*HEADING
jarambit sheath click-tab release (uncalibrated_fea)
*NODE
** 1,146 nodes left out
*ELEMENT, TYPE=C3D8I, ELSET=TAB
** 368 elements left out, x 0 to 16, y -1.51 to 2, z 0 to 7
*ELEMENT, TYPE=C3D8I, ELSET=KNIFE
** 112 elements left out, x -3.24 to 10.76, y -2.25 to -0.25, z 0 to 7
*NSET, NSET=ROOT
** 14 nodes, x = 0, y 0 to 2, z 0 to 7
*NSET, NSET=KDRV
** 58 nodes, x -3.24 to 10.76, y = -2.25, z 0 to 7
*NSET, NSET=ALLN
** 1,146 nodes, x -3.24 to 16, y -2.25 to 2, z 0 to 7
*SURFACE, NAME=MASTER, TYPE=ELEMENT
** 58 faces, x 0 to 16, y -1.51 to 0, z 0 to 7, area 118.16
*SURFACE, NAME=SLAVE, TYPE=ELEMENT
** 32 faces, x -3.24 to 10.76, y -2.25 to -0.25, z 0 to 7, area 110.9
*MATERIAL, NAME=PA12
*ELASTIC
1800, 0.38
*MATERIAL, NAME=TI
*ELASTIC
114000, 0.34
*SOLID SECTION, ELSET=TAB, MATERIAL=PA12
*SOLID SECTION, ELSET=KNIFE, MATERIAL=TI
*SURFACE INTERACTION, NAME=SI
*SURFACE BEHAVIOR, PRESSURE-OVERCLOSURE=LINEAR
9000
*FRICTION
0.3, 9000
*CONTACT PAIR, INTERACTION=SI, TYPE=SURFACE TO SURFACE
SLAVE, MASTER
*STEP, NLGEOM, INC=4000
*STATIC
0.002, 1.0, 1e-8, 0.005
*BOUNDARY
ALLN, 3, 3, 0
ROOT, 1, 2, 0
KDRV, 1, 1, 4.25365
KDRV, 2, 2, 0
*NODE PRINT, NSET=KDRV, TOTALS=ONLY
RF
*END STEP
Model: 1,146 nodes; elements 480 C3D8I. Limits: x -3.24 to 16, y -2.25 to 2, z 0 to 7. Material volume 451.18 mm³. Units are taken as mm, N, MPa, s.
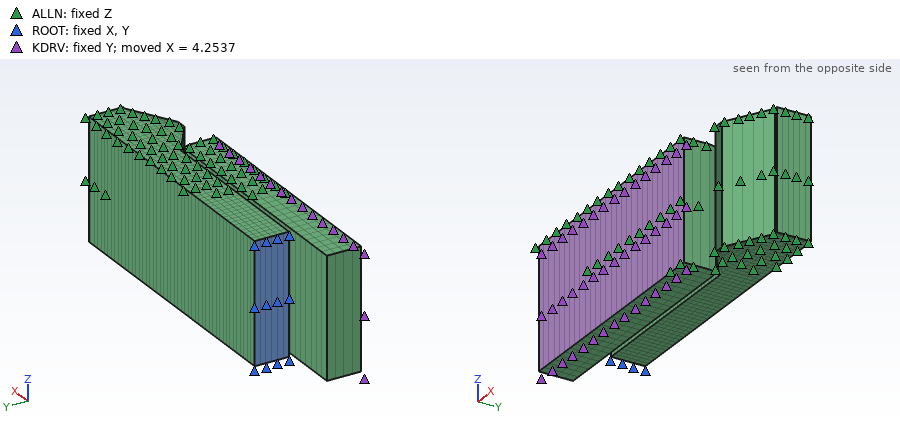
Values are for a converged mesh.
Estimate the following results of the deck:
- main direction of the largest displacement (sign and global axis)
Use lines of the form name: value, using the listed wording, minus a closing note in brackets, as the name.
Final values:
main direction of the largest displacement: +X
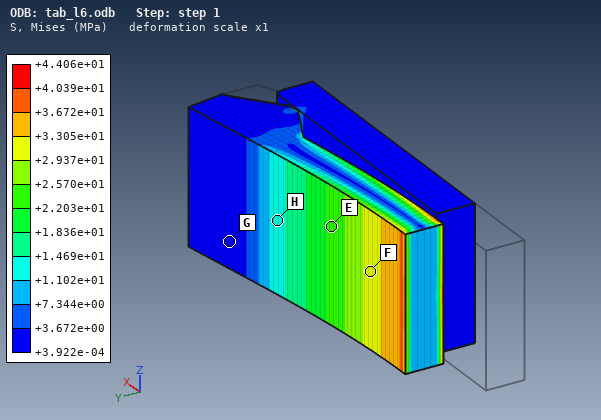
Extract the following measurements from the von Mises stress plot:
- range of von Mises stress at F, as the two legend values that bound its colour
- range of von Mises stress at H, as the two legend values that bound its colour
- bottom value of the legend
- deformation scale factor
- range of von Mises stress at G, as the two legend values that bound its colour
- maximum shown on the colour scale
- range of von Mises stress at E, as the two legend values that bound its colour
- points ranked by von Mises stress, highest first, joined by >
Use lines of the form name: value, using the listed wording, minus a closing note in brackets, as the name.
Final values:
range of von Mises stress at F, as the two legend values that bound its colour: +2.937e+01 to +3.305e+01 MPa
range of von Mises stress at H, as the two legend values that bound its colour: +1.102e+01 to +1.469e+01 MPa
bottom value of the legend: +3.922e-04 MPa
deformation scale factor: 1
range of von Mises stress at G, as the two legend values that bound its colour: +3.922e-04 to +3.672e+00 MPa
maximum shown on the colour scale: +4.406e+01 MPa
range of von Mises stress at E, as the two legend values that bound its colour: +2.203e+01 to +2.570e+01 MPa
points ranked by von Mises stress, highest first, joined by >: F > E > H > G
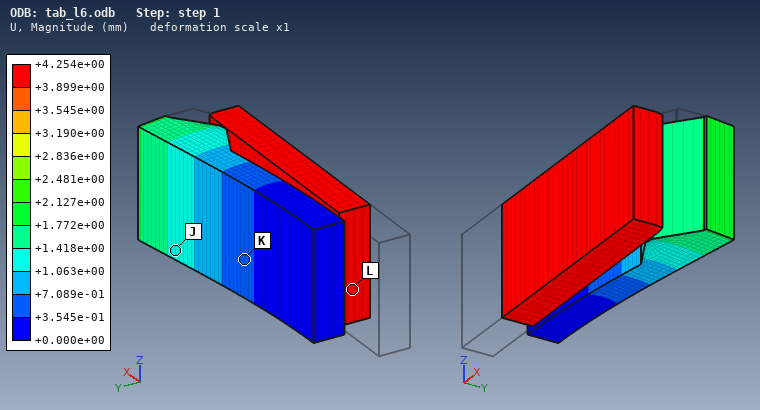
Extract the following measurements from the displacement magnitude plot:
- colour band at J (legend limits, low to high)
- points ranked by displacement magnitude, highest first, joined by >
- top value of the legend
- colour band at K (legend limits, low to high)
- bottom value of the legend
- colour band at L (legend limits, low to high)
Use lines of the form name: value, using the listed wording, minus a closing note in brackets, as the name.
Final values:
colour band at J: +1.063e+00 to +1.418e+00 mm
points ranked by displacement magnitude, highest first, joined by >: L > J > K
top value of the legend: +4.254e+00 mm
colour band at K: +3.545e-01 to +7.089e-01 mm
bottom value of the legend: +0.000e+00 mm
colour band at L: +3.899e+00 to +4.254e+00 mm
